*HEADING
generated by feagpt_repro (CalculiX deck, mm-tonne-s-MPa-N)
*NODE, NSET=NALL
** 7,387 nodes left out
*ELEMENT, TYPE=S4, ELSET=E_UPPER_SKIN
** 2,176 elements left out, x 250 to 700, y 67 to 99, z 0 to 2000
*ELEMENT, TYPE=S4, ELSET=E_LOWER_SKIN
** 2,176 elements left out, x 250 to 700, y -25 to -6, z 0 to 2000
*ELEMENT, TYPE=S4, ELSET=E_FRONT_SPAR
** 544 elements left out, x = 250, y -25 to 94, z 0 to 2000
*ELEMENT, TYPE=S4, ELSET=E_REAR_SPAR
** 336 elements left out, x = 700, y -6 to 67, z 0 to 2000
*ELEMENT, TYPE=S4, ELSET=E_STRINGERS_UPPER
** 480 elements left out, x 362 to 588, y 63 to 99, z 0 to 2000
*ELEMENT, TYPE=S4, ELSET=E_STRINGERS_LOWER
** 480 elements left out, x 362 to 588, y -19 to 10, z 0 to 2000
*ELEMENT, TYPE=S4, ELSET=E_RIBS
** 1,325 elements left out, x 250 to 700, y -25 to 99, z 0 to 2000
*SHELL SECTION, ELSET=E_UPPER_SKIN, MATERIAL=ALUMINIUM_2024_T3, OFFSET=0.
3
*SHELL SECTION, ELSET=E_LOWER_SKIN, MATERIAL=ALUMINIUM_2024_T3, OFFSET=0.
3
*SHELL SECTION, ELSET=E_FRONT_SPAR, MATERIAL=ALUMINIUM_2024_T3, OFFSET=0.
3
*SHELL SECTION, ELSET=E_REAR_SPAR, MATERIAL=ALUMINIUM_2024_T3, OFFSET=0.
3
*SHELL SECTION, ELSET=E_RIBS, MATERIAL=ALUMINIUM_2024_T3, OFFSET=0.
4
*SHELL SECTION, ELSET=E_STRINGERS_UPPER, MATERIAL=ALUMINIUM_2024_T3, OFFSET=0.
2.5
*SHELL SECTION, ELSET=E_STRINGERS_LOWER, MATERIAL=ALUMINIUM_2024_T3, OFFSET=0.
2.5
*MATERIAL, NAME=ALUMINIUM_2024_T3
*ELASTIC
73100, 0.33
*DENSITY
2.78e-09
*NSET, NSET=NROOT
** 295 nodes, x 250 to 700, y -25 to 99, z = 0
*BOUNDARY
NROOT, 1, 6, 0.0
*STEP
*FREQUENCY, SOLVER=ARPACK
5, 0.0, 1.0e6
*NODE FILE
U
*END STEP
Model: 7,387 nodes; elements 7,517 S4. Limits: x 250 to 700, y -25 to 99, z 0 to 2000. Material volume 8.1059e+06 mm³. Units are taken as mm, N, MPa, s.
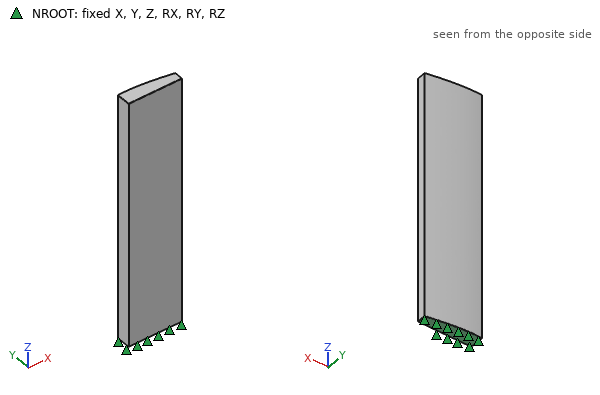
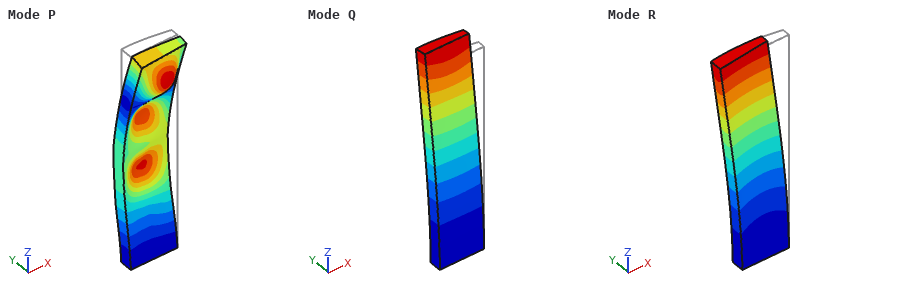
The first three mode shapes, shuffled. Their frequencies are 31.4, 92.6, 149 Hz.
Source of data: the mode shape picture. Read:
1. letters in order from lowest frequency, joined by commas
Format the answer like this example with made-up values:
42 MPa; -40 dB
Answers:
Q, R, P
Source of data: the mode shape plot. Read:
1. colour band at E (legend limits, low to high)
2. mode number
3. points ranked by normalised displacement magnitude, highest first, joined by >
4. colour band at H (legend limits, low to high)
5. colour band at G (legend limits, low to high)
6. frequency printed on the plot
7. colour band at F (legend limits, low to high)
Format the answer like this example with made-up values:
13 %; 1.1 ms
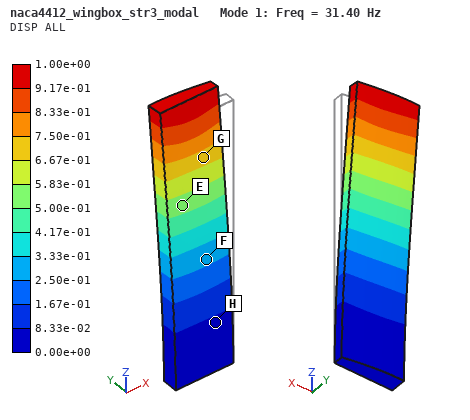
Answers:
5.00e-01 to 5.83e-01; 1; G > E > F > H; 0.00e+00 to 8.33e-02; 6.67e-01 to 7.50e-01; 31.40 Hz; 2.50e-01 to 3.33e-01
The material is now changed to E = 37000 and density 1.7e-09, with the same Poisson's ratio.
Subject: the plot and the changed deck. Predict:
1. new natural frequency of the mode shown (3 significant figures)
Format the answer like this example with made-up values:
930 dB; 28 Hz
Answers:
28.6 Hz
